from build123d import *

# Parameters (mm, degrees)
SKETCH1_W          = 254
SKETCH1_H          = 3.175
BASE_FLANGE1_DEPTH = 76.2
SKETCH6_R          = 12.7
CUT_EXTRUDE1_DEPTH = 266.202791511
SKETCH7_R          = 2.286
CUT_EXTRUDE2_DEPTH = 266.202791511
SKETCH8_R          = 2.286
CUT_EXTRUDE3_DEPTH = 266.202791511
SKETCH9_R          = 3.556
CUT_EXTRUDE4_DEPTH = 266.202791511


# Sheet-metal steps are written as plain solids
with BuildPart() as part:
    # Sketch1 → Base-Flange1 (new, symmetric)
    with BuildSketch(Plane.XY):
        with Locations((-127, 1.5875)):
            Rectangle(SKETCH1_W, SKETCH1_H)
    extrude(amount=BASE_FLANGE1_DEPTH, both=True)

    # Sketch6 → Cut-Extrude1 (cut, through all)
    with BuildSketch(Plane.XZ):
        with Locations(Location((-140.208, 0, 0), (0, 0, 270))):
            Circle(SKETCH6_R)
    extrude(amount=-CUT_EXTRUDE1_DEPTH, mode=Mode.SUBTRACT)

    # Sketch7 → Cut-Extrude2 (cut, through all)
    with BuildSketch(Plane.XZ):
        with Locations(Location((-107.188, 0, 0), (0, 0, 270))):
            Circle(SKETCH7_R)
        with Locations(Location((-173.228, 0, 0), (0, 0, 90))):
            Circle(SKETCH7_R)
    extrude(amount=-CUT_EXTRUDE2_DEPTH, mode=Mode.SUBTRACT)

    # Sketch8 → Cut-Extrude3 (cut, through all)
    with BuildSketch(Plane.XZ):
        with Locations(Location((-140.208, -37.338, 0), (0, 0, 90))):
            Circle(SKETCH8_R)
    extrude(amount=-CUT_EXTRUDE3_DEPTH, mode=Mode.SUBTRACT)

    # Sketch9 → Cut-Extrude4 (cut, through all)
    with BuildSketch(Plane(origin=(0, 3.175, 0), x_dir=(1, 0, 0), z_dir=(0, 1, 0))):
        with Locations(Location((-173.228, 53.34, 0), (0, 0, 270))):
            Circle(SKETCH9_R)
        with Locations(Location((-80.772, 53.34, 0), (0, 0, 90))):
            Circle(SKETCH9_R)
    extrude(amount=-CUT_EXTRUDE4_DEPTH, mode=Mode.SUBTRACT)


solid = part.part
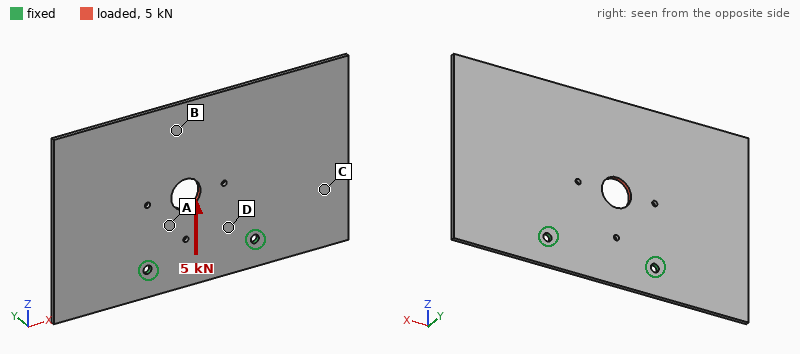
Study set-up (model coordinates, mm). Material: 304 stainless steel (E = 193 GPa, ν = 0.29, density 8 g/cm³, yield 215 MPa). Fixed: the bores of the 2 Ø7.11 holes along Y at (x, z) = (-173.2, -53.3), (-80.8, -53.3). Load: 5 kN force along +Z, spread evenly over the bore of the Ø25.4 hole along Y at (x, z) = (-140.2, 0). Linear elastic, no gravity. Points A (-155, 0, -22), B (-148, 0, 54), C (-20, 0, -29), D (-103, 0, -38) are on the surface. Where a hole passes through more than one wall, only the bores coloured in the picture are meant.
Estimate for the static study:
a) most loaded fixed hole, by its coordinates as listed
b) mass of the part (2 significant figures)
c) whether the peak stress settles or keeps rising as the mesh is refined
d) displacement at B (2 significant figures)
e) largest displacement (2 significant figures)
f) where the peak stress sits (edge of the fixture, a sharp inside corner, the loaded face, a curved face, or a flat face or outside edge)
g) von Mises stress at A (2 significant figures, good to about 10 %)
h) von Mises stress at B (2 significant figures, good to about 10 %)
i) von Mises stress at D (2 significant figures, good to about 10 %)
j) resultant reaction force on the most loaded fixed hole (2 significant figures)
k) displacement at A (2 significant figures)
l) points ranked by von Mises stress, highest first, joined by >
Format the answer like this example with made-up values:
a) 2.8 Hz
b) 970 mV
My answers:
a) (-173.2, -53.3)
b) 970 g
c) keeps rising
d) 7.2 µm
e) 9.0 µm
f) edge of the fixture
g) 21 MPa
h) 5.5 MPa
i) 12 MPa
j) 3.2 kN
k) 5.3 µm
l) A > D > B > C
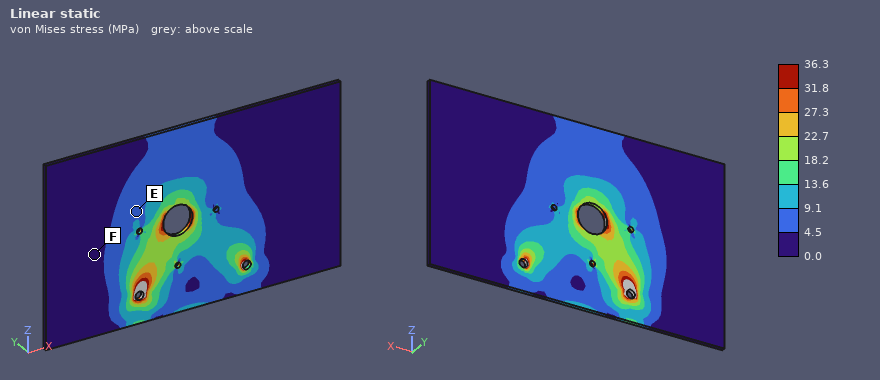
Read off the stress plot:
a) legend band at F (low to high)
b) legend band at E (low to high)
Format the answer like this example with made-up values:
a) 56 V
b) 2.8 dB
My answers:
a) 0.0 to 4.5 MPa
b) 4.5 to 9.1 MPa
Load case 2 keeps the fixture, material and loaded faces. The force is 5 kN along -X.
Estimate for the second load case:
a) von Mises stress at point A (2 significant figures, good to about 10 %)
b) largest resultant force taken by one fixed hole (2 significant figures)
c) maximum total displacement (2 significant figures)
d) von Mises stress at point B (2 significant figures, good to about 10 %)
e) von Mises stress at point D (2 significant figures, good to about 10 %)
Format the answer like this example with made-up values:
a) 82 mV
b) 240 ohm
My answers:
a) 22 MPa
b) 3.8 kN
c) 31 µm
d) 6.0 MPa
e) 24 MPa
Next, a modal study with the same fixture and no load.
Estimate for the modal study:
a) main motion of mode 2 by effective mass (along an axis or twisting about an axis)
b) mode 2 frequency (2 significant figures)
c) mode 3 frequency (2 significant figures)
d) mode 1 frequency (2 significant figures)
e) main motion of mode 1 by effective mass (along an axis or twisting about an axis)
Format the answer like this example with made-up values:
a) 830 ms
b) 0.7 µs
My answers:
a) twisting about Z
b) 170 Hz
c) 300 Hz
d) 120 Hz
e) along Y
